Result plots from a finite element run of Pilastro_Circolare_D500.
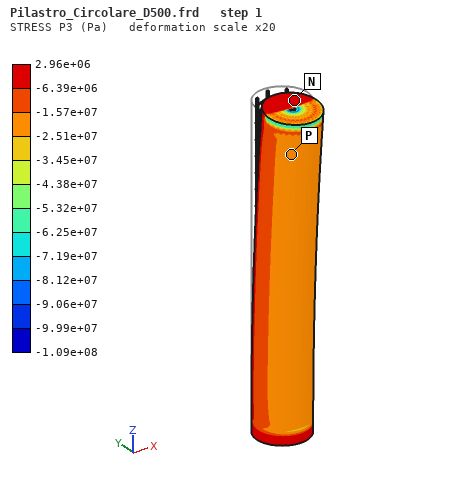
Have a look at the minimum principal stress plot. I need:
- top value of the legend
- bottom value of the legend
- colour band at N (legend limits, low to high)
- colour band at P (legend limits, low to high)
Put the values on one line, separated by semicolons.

2.96e+06 Pa; -1.09e+08 Pa; -6.39e+06 to 2.96e+06 Pa; -2.51e+07 to -1.57e+07 Pa
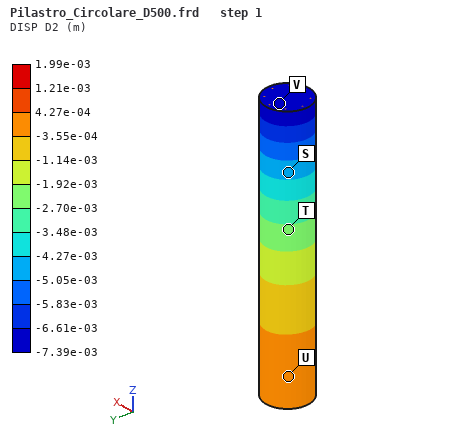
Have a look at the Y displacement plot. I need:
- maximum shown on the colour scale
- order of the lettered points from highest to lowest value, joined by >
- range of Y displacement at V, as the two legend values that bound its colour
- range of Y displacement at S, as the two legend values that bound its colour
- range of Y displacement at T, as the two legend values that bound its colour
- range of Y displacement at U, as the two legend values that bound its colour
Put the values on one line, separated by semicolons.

1.99e-03 m; U > T > S > V; -7.39e-03 to -6.61e-03 m; -5.05e-03 to -4.27e-03 m; -2.70e-03 to -1.92e-03 m; -3.55e-04 to 4.27e-04 m
